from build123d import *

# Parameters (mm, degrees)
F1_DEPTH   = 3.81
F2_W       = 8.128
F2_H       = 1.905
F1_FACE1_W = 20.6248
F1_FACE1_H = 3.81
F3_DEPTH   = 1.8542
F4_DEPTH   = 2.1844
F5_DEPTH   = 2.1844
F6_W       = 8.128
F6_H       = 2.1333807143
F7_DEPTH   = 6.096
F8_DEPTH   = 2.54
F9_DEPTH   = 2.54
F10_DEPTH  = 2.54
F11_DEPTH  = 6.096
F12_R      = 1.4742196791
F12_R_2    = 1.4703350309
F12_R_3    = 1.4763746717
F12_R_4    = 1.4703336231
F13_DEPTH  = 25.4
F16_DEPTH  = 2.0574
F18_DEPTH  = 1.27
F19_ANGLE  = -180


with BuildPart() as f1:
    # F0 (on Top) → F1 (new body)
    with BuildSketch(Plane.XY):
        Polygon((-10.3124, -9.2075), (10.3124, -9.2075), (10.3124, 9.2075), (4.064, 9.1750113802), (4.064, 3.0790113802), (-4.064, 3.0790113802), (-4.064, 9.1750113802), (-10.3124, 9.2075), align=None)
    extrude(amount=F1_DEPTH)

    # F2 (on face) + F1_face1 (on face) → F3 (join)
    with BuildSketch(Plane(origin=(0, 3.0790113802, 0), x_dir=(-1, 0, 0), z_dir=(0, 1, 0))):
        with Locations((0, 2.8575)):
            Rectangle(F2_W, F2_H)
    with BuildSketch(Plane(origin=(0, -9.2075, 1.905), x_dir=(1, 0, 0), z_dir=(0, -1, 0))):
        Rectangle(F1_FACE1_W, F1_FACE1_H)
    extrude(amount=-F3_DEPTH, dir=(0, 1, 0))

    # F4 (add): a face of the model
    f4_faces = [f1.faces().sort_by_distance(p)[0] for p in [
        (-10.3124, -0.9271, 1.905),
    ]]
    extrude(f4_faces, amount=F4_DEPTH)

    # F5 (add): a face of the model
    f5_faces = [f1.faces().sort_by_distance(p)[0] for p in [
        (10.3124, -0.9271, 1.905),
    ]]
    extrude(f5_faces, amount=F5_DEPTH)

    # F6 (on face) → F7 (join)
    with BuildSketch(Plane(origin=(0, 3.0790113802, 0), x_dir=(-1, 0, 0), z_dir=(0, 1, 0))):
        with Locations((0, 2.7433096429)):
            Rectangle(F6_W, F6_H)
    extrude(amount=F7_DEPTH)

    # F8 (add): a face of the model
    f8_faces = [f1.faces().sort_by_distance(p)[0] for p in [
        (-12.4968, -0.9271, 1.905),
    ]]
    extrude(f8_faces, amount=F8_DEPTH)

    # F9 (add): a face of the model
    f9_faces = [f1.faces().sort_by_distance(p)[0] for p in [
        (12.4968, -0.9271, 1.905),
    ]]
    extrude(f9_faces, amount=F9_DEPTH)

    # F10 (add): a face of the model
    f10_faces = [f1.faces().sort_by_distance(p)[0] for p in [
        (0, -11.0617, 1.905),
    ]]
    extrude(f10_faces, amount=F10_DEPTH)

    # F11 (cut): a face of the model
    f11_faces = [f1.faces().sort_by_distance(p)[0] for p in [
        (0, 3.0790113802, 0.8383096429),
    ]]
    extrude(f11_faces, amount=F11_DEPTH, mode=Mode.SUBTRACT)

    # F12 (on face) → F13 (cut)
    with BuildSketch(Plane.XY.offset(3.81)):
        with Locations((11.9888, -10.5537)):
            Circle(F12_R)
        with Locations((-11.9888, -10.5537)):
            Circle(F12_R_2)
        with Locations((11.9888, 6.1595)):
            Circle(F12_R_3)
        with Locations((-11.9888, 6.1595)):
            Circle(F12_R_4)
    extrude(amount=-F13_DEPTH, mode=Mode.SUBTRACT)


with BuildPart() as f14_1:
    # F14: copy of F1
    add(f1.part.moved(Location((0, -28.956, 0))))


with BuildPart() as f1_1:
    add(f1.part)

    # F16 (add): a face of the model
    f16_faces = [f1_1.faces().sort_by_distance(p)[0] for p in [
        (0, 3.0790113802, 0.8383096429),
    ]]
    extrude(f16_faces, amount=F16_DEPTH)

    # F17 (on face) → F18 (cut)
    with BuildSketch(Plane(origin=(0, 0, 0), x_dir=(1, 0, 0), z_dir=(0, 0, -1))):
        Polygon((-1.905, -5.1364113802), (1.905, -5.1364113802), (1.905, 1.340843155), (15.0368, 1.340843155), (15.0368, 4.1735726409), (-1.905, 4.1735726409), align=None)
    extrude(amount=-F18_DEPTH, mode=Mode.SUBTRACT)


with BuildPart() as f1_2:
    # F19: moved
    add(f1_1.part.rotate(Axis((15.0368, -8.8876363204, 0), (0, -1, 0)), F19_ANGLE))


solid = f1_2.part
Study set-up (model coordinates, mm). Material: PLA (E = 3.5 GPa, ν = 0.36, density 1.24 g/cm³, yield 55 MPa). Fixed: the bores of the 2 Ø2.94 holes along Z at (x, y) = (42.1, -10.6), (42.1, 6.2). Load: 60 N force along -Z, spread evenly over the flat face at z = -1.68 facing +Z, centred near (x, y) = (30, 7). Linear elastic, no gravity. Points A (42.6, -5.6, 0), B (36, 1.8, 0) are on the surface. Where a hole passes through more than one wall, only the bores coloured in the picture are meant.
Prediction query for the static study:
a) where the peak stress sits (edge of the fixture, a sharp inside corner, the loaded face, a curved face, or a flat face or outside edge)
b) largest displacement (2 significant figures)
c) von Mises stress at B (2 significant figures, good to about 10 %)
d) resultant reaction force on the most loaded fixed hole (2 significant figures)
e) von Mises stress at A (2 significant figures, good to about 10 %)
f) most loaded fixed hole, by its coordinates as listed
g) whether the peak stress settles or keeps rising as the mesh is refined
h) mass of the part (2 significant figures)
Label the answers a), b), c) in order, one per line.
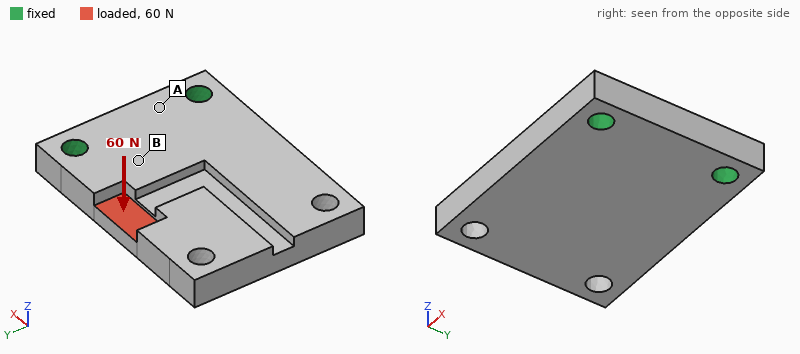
a) edge of the fixture
b) 0.44 mm
c) 8.8 MPa
d) 63 N
e) 4.1 MPa
f) (42.1, 6.2)
g) keeps rising
h) 2.9 g
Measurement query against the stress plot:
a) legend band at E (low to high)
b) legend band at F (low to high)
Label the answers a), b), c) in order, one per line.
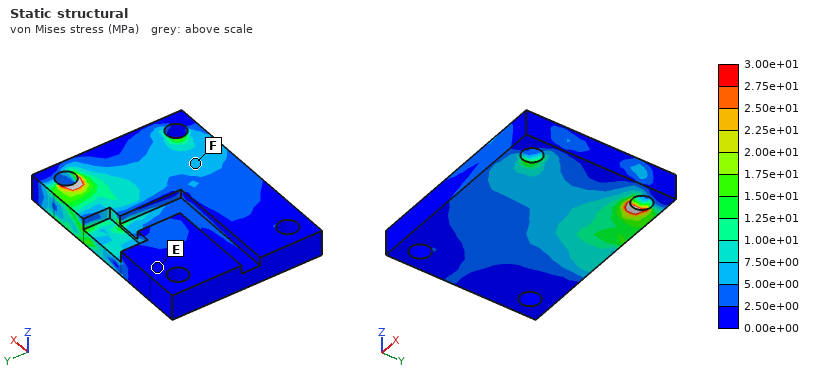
a) 0.00e+00 to 2.50e+00 MPa
b) 5.00e+00 to 7.50e+00 MPa
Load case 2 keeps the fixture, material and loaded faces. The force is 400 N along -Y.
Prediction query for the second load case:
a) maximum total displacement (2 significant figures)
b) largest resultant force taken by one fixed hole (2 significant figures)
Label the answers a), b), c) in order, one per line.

a) 0.17 mm
b) 330 N
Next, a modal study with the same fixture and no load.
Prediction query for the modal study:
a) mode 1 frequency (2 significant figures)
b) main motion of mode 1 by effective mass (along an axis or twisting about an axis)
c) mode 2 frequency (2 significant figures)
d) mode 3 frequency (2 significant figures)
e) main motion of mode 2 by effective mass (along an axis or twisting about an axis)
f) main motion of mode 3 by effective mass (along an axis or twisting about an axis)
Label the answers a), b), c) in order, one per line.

a) 1300 Hz
b) along Z
c) 3400 Hz
d) 5900 Hz
e) twisting about X
f) along Y
